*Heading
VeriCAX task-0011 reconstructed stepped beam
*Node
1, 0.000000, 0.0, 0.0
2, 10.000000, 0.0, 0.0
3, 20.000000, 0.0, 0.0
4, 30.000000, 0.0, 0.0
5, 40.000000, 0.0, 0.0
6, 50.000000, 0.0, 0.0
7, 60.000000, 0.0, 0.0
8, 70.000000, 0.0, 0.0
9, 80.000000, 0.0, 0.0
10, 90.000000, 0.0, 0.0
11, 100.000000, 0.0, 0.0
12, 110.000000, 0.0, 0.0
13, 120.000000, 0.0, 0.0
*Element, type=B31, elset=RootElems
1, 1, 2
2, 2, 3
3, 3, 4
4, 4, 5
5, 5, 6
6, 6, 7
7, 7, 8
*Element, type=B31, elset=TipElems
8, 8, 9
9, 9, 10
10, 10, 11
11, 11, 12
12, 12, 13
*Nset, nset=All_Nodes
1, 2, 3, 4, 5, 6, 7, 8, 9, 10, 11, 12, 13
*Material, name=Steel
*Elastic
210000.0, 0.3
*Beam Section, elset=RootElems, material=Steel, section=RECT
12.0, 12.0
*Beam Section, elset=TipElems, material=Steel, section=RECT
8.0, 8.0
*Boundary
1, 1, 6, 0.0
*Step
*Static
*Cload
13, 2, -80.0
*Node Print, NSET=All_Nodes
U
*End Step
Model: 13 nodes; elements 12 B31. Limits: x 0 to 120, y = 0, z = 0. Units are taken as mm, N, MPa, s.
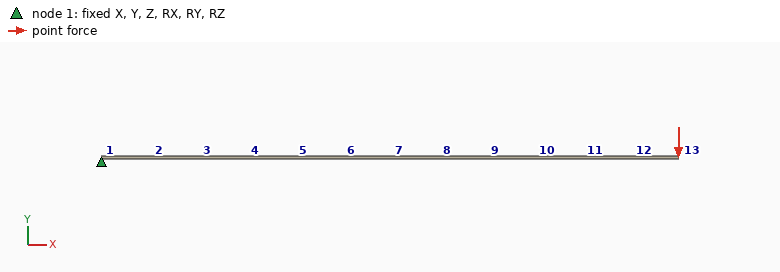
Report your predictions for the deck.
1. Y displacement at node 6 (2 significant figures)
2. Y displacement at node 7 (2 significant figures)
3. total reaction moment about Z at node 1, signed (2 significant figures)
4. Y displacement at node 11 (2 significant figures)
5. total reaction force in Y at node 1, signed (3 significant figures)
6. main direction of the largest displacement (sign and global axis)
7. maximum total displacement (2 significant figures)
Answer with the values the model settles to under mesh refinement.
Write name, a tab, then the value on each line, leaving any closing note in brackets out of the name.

Y displacement at node 6	-0.029 mm
Y displacement at node 7	-0.040 mm
total reaction moment about Z at node 1, signed	9600 N·mm
Y displacement at node 11	-0.11 mm
total reaction force in Y at node 1, signed	80.0 N
main direction of the largest displacement	-Y
maximum total displacement	0.17 mm
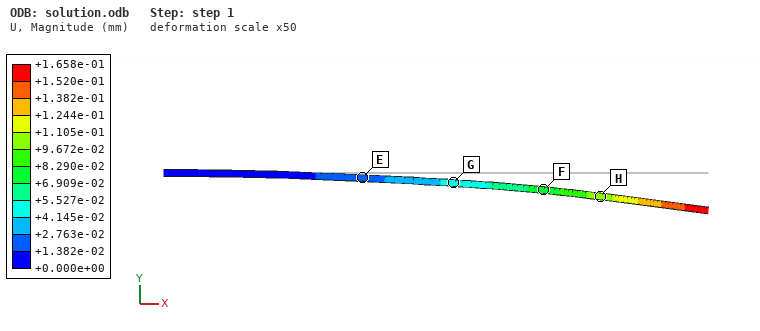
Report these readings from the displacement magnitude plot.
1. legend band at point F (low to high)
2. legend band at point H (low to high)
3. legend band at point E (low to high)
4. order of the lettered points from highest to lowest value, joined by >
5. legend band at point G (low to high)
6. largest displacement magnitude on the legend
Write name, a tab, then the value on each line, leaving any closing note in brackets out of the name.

legend band at point F	+6.909e-02 to +8.290e-02 mm
legend band at point H	+9.672e-02 to +1.105e-01 mm
legend band at point E	+1.382e-02 to +2.763e-02 mm
order of the lettered points from highest to lowest value, joined by >	H > F > G > E
legend band at point G	+4.145e-02 to +5.527e-02 mm
largest displacement magnitude on the legend	+1.658e-01 mm
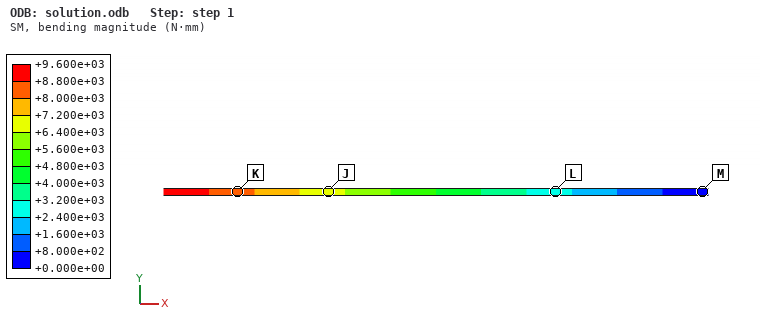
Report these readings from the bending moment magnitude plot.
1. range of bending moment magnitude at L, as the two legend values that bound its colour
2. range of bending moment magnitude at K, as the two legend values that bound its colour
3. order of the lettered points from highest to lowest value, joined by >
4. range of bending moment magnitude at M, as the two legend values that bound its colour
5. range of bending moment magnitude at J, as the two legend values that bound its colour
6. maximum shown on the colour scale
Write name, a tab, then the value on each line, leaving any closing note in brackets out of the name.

range of bending moment magnitude at L, as the two legend values that bound its colour	+2.400e+03 to +3.200e+03 N·mm
range of bending moment magnitude at K, as the two legend values that bound its colour	+8.000e+03 to +8.800e+03 N·mm
order of the lettered points from highest to lowest value, joined by >	K > J > L > M
range of bending moment magnitude at M, as the two legend values that bound its colour	+0.000e+00 to +8.000e+02 N·mm
range of bending moment magnitude at J, as the two legend values that bound its colour	+6.400e+03 to +7.200e+03 N·mm
maximum shown on the colour scale	+9.600e+03 N·mm
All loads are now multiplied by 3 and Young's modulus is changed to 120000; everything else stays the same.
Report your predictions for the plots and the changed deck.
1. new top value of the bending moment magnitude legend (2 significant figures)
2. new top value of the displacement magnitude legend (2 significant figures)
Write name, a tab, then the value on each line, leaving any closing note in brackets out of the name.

new top value of the bending moment magnitude legend	29000 N·mm
new top value of the displacement magnitude legend	0.87 mm
